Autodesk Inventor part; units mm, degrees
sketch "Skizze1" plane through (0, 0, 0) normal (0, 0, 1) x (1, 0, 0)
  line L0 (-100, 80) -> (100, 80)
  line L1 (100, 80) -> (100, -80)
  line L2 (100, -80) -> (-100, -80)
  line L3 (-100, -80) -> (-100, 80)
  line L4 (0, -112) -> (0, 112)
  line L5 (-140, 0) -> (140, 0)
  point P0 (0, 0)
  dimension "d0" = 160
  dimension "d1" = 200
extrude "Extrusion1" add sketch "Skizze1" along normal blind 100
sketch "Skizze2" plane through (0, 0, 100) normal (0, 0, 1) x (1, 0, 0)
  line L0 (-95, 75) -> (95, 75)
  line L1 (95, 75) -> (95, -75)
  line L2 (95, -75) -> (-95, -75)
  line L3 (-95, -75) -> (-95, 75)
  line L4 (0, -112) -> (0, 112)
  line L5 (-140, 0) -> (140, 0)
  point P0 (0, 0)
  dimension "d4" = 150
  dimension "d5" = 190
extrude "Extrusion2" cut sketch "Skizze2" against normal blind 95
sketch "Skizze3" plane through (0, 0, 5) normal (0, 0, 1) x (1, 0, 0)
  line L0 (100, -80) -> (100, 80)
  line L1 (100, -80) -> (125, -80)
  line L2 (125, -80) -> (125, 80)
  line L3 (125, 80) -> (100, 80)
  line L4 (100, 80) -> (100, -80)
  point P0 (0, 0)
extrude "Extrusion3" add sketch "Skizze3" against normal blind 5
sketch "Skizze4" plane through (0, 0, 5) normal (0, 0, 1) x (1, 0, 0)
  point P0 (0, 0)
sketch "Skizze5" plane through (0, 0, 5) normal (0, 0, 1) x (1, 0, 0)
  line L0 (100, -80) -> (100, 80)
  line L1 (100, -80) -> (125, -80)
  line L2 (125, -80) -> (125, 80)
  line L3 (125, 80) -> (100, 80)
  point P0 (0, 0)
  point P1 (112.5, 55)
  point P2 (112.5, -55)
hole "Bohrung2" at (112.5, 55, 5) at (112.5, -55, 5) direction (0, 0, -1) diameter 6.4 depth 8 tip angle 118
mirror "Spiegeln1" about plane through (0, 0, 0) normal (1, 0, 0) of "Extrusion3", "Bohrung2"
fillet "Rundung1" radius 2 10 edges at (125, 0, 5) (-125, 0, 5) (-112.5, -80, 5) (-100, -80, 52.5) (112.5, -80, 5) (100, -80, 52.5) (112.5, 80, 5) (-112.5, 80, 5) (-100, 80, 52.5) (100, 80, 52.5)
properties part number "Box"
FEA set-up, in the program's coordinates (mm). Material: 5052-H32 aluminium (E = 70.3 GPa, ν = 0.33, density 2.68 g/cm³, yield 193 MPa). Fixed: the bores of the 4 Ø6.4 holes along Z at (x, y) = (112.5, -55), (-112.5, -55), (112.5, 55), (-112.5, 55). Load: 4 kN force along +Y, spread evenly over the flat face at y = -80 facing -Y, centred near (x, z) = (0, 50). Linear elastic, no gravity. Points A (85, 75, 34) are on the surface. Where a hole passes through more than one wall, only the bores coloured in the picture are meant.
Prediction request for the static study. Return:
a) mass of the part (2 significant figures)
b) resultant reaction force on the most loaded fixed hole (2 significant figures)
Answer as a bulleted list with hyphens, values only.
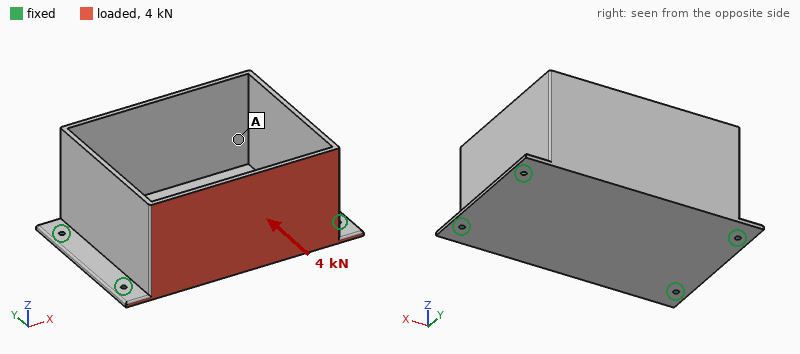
- 1.4 kg
- 1.5 kN
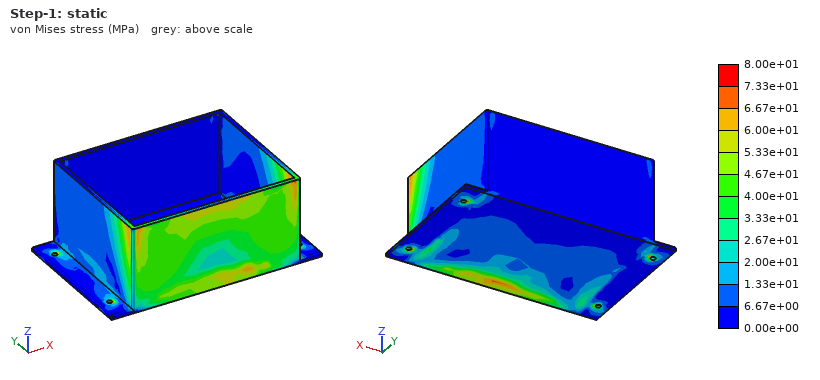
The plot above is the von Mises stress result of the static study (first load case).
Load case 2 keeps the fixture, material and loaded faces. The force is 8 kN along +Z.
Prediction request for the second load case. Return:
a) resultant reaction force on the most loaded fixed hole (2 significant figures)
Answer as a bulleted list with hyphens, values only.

- 5.2 kN
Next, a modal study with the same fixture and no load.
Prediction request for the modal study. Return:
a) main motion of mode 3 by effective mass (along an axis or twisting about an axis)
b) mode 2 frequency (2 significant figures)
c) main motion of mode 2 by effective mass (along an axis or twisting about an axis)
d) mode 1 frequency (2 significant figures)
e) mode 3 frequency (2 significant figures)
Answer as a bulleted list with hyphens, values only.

- along X
- 760 Hz
- along Y
- 700 Hz
- 1000 Hz
